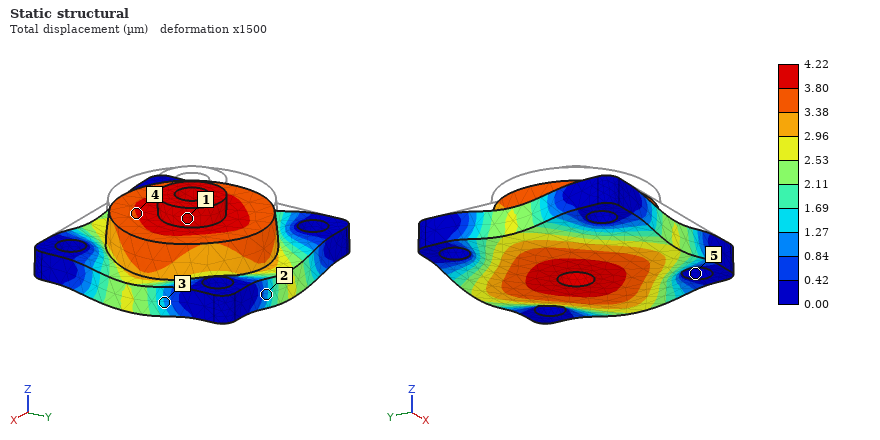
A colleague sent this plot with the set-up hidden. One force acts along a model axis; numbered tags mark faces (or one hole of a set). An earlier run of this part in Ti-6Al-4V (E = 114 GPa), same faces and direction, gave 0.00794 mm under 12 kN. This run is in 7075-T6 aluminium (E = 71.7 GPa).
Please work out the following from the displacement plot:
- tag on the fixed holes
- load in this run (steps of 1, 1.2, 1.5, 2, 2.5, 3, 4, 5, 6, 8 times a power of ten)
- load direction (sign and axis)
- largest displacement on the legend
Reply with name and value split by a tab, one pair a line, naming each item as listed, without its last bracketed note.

tag on the fixed holes	5
load in this run	4 kN
load direction	-Z
largest displacement on the legend	4.22 µm
